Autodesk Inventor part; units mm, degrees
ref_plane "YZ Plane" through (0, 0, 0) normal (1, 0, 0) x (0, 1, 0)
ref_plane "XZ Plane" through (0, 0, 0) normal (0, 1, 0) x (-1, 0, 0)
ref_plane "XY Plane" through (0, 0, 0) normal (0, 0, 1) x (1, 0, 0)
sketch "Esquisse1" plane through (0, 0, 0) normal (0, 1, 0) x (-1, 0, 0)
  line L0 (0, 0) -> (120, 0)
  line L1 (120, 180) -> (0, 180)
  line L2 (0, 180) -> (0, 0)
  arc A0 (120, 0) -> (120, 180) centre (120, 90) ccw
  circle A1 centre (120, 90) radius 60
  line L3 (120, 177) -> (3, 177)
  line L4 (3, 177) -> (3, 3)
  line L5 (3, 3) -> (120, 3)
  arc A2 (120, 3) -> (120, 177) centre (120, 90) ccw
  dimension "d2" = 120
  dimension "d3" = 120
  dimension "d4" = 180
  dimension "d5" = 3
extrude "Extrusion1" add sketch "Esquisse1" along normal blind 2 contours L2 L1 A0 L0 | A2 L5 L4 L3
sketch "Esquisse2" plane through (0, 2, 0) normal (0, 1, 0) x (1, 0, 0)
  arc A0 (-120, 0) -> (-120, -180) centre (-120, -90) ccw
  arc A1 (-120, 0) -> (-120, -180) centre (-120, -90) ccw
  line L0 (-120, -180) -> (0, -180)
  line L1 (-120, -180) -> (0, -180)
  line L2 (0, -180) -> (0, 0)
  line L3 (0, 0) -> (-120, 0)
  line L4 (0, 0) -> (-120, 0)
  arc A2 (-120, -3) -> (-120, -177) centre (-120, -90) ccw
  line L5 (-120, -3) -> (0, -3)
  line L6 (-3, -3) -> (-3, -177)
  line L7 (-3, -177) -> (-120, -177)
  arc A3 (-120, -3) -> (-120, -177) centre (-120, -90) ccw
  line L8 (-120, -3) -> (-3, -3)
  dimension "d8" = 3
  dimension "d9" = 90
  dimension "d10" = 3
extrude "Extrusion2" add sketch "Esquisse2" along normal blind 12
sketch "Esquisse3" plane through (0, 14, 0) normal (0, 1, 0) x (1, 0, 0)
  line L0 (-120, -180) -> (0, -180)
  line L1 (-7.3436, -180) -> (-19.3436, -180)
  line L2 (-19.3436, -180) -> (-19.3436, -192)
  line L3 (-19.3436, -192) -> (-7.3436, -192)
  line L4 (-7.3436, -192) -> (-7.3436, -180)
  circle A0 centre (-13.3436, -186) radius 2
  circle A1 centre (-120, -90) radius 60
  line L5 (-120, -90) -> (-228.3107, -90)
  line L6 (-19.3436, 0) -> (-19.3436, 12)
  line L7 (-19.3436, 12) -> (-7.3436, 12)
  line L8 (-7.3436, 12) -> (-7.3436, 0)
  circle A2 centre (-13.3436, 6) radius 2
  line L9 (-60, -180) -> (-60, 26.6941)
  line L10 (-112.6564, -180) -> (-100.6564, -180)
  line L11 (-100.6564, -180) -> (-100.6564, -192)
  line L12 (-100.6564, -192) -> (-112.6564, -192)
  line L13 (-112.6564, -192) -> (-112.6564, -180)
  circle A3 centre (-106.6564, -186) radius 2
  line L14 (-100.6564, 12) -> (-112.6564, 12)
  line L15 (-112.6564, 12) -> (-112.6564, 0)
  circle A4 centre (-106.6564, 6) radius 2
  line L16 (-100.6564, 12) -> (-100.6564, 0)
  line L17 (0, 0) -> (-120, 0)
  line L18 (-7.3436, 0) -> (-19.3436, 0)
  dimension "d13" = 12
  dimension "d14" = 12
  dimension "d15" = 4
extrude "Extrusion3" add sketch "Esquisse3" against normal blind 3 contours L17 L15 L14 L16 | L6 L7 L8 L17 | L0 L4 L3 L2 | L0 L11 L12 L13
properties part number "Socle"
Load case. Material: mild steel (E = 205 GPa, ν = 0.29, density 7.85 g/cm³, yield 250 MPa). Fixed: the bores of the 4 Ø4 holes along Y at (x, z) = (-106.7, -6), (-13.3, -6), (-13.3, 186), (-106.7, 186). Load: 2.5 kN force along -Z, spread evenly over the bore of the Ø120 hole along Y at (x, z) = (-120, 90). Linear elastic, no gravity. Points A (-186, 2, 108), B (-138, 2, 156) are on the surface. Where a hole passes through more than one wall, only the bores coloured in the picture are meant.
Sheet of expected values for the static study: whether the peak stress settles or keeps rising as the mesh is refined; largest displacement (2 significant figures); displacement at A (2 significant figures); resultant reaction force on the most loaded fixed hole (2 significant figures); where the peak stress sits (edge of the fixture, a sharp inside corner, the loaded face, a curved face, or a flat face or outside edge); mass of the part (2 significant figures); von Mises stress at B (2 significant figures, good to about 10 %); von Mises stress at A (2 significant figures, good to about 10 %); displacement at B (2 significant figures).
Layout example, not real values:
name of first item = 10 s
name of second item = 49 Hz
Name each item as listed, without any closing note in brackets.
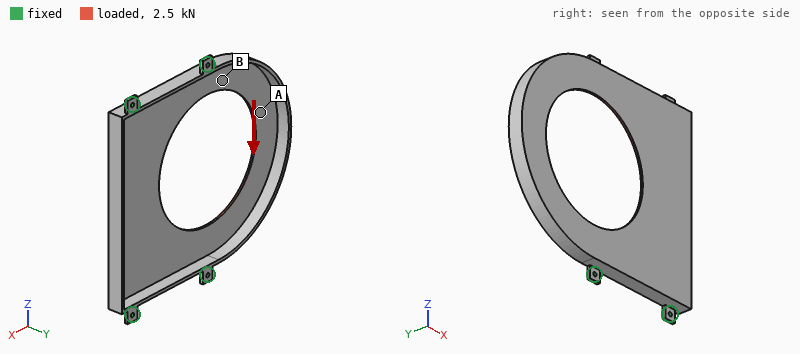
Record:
whether the peak stress settles or keeps rising as the mesh is refined = keeps rising
largest displacement = 0.13 mm
displacement at A = 0.083 mm
resultant reaction force on the most loaded fixed hole = 890 N
where the peak stress sits = edge of the fixture
mass of the part = 570 g
von Mises stress at B = 35 MPa
von Mises stress at A = 14 MPa
displacement at B = 0.086 mm
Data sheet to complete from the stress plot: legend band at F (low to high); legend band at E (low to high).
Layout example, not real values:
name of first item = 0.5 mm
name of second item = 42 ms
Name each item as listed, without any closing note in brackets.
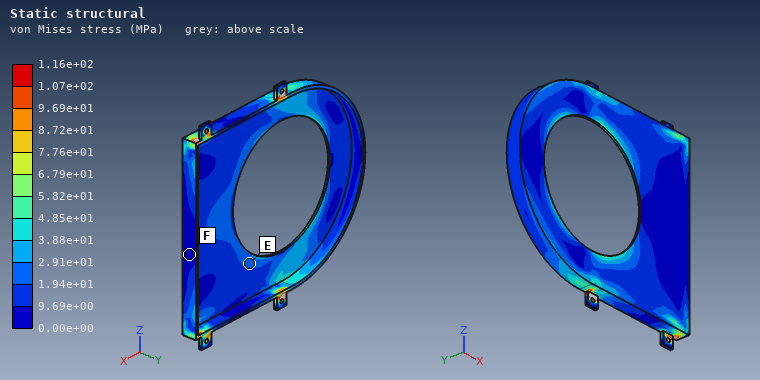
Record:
legend band at F = 0.00e+00 to 9.69e+00 MPa
legend band at E = 1.94e+01 to 2.91e+01 MPa
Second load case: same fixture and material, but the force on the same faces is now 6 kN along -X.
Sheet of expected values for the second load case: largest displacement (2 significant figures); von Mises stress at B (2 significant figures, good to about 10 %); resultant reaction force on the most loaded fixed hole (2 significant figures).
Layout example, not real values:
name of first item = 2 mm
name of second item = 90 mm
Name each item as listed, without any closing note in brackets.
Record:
largest displacement = 0.17 mm
von Mises stress at B = 30 MPa
resultant reaction force on the most loaded fixed hole = 1.6 kN
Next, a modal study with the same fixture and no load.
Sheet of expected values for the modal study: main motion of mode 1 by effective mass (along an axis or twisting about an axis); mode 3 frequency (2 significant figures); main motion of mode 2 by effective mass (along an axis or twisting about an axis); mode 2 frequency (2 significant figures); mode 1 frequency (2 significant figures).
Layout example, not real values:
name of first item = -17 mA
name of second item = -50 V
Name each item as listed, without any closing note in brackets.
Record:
main motion of mode 1 by effective mass = along Y
mode 3 frequency = 970 Hz
main motion of mode 2 by effective mass = along Y
mode 2 frequency = 560 Hz
mode 1 frequency = 440 Hz
